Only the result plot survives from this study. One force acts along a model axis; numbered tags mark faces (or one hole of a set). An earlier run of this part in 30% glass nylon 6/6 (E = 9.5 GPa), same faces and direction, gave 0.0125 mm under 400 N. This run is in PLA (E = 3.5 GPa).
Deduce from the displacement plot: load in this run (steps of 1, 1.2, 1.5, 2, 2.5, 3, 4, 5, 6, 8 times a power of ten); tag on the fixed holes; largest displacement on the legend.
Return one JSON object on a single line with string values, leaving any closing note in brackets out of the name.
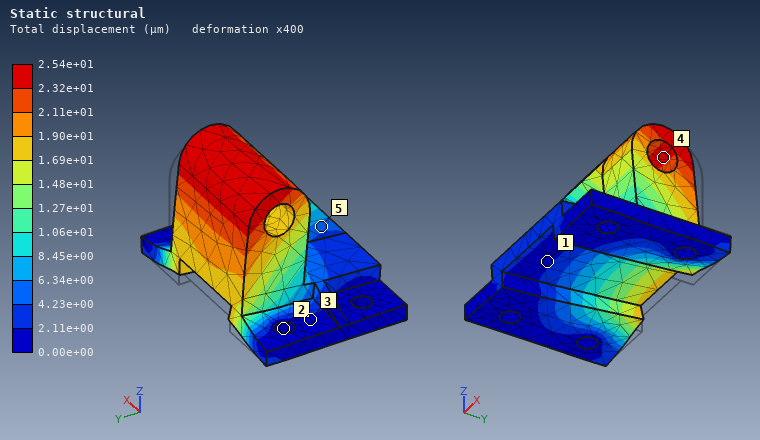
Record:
{"load in this run": "300 N", "tag on the fixed holes": "2", "largest displacement on the legend": "2.54e+01 µm"}
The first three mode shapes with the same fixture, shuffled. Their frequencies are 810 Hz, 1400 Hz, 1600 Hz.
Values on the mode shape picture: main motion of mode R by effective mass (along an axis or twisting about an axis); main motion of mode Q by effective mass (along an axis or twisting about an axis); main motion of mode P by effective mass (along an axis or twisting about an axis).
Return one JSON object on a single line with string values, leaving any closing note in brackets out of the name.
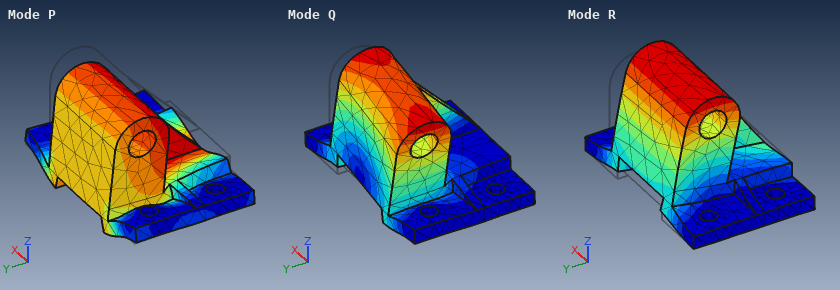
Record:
{"main motion of mode R by effective mass": "along Y", "main motion of mode Q by effective mass": "along X", "main motion of mode P by effective mass": "along Z"}
